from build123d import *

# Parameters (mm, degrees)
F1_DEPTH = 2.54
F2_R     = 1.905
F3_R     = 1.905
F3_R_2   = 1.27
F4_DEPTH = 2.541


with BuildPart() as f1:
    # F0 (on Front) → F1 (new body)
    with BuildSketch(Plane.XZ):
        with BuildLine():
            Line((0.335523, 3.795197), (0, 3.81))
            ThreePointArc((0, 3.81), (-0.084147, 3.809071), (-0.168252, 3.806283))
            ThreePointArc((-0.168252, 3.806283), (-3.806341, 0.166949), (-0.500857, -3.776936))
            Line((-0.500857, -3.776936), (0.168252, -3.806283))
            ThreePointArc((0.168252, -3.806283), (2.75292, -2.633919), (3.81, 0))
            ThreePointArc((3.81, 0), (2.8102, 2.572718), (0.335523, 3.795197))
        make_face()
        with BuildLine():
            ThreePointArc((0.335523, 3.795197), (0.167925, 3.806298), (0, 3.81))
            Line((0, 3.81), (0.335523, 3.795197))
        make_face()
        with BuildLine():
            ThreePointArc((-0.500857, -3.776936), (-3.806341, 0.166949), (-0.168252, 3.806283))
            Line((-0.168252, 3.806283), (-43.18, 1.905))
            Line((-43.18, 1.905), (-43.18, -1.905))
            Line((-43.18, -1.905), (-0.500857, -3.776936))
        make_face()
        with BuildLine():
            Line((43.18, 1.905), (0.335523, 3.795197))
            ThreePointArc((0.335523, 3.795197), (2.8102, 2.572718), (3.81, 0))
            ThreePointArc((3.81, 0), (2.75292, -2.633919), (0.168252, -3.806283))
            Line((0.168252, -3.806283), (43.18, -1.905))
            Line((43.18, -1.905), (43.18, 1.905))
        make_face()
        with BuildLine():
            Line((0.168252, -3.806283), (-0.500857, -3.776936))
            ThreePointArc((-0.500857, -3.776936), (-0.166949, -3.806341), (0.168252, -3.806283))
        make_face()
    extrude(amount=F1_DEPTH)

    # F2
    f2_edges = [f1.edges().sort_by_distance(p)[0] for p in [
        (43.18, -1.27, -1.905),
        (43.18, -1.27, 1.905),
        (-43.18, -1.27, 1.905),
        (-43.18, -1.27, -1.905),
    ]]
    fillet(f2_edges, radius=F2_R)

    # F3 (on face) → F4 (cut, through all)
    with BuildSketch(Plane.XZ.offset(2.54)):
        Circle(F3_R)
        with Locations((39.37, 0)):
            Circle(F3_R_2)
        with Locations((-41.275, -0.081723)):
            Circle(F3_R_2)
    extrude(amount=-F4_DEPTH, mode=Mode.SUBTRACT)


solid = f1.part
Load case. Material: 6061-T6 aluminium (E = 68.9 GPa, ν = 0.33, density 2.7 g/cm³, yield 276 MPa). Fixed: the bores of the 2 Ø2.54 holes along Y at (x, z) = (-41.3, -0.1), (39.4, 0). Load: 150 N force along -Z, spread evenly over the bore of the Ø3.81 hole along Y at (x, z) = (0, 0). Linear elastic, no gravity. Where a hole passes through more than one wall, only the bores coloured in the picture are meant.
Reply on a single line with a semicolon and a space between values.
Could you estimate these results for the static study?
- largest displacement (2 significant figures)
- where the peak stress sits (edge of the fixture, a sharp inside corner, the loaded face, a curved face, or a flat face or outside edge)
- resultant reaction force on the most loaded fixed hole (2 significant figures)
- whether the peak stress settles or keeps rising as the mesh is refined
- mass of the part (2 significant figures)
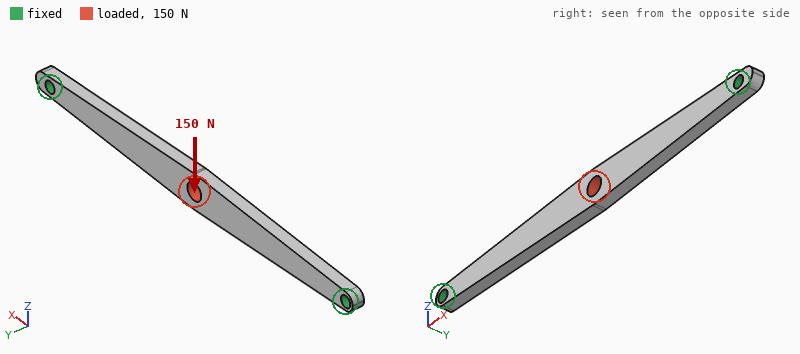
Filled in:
0.16 mm; edge of the fixture; 78 N; keeps rising; 3.2 g
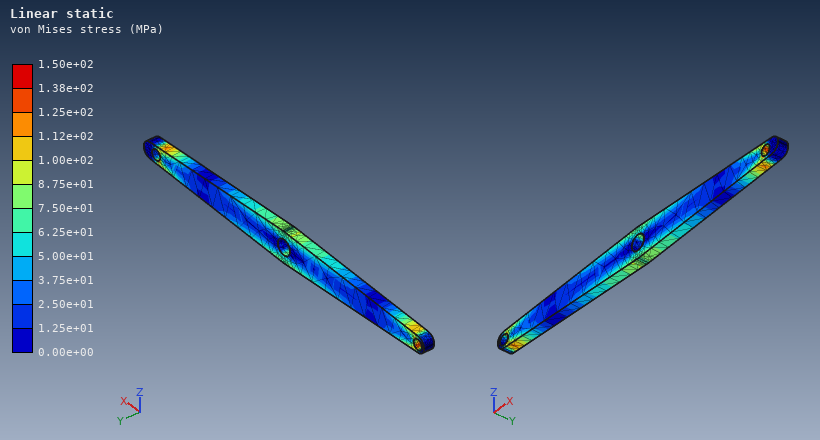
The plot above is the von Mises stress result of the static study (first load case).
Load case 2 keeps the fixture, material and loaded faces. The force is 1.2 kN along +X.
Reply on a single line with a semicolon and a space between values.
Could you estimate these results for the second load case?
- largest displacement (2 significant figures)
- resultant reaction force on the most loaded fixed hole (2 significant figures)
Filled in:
24 µm; 620 N
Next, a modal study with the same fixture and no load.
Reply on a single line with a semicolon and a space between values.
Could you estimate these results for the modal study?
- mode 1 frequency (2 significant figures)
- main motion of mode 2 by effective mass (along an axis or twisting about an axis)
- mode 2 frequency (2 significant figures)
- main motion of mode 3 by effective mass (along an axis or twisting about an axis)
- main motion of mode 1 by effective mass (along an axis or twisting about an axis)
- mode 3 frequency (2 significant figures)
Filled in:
1900 Hz; along Z; 3900 Hz; twisting about Z; along Y; 5500 Hz
